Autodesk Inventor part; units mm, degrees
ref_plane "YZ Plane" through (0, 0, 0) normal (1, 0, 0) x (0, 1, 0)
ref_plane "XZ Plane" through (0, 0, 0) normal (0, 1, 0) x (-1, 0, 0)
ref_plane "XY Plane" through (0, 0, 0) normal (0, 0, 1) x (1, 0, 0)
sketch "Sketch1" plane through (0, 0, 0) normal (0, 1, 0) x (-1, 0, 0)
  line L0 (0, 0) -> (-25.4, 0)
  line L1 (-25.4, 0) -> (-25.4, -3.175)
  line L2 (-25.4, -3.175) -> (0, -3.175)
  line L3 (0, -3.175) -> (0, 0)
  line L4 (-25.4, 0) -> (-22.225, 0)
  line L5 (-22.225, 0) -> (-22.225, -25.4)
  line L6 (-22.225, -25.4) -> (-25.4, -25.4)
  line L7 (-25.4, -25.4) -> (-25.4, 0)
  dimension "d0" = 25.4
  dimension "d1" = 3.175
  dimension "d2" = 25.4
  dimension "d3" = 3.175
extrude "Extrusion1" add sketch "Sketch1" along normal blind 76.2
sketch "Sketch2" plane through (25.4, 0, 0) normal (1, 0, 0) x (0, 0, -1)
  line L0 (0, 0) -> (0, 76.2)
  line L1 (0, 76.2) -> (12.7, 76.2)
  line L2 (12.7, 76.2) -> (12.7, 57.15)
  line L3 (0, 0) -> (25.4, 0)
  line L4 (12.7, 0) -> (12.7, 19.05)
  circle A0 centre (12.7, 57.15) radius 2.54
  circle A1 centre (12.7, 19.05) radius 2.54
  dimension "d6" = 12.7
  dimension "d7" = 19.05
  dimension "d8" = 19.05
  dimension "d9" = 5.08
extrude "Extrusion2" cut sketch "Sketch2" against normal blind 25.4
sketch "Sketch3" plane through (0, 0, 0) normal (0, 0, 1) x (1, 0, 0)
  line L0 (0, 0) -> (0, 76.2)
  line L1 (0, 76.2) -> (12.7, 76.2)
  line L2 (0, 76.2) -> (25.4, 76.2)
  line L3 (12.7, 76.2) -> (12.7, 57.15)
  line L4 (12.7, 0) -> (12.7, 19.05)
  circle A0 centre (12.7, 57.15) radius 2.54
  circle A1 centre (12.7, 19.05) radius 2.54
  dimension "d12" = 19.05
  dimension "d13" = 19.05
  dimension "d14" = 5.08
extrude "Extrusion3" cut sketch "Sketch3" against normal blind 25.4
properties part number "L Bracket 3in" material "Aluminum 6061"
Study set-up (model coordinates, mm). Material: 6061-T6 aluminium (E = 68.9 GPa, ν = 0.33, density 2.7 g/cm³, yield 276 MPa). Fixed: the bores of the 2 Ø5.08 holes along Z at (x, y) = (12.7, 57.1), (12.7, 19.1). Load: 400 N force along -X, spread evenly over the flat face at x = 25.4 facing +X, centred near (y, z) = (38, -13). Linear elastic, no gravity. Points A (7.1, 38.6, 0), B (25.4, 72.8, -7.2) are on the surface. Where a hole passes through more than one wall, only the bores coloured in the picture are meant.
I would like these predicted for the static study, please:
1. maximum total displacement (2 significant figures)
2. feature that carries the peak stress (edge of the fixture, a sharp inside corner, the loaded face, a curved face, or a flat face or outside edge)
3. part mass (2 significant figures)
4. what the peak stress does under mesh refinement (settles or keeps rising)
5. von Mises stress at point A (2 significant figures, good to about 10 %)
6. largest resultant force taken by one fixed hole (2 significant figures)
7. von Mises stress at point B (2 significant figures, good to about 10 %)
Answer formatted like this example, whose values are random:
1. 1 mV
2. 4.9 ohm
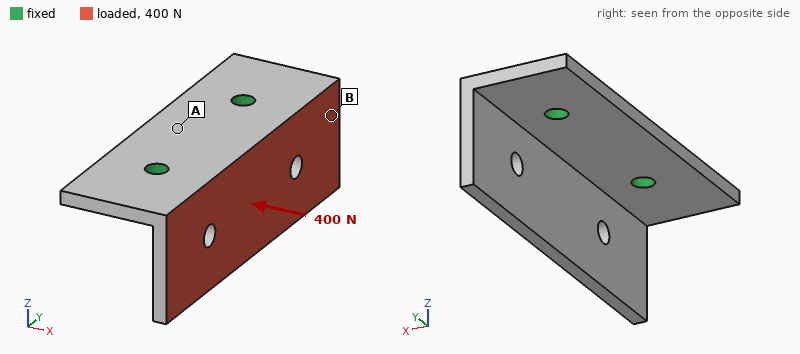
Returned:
1. 0.13 mm
2. edge of the fixture
3. 30 g
4. keeps rising
5. 7.0 MPa
6. 200 N
7. 19 MPa
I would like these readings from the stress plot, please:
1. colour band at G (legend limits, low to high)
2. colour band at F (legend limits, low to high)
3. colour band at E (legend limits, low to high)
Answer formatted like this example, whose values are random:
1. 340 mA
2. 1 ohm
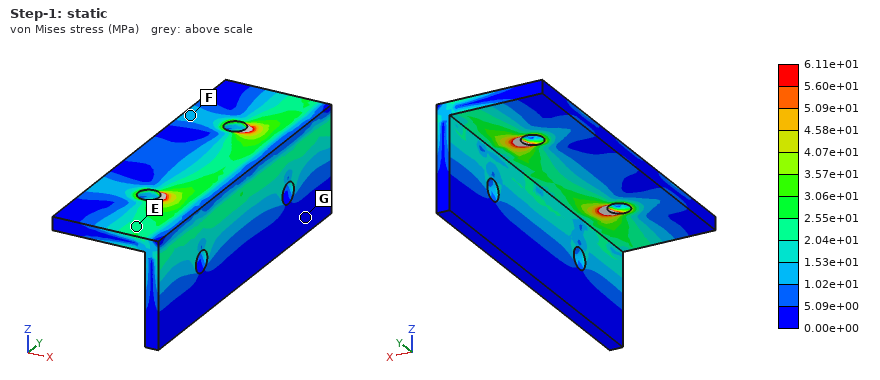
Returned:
1. 0.00e+00 to 5.09e+00 MPa
2. 1.02e+01 to 1.53e+01 MPa
3. 2.04e+01 to 2.55e+01 MPa
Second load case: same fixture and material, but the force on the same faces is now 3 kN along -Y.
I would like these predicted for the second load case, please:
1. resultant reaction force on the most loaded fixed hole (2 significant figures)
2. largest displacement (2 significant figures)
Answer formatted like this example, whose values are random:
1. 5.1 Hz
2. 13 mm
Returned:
1. 1.9 kN
2. 0.13 mm
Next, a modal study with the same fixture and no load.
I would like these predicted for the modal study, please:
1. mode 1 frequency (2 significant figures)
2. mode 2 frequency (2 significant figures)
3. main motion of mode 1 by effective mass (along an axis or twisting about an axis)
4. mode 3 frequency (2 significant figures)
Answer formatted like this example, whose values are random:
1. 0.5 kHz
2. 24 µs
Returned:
1. 2600 Hz
2. 3600 Hz
3. along X
4. 6600 Hz
